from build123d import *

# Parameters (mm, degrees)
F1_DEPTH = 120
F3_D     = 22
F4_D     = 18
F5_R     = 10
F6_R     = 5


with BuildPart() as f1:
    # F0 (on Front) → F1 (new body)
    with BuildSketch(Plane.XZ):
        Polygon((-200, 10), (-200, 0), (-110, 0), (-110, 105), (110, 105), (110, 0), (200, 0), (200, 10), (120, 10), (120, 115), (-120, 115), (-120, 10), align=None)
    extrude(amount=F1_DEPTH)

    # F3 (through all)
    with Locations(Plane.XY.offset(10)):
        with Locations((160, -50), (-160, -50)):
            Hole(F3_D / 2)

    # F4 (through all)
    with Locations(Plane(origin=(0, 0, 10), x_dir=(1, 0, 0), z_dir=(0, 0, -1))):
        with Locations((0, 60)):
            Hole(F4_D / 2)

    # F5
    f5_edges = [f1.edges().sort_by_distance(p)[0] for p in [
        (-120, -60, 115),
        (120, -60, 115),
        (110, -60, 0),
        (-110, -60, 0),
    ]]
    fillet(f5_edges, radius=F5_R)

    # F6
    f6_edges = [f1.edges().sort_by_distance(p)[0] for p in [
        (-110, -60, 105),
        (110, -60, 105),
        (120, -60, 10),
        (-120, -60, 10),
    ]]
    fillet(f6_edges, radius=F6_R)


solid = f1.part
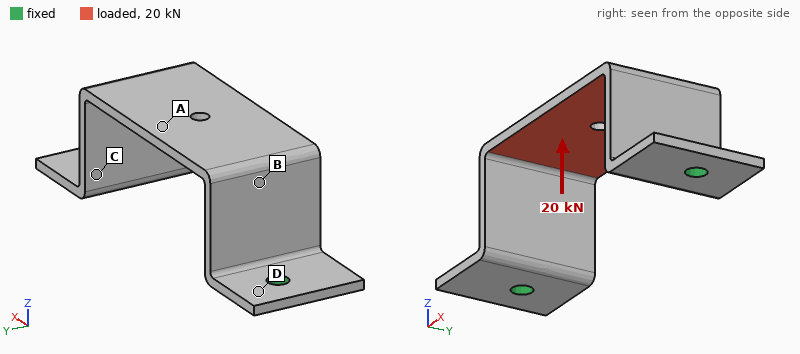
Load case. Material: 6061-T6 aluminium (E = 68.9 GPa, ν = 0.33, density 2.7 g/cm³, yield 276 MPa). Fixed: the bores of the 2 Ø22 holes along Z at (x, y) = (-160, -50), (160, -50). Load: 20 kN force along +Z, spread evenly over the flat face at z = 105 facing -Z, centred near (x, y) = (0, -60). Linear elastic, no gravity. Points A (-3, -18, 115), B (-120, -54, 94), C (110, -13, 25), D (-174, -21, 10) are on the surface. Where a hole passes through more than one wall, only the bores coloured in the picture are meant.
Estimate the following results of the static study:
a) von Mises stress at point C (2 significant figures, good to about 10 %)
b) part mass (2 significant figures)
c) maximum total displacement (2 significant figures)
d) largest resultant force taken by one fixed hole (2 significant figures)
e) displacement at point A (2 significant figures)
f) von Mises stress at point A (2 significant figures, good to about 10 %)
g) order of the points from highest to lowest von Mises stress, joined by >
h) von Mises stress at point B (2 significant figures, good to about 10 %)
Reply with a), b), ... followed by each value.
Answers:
a) 36 MPa
b) 1.9 kg
c) 1.9 mm
d) 11 kN
e) 1.6 mm
f) 140 MPa
g) A > B > C > D
h) 120 MPa
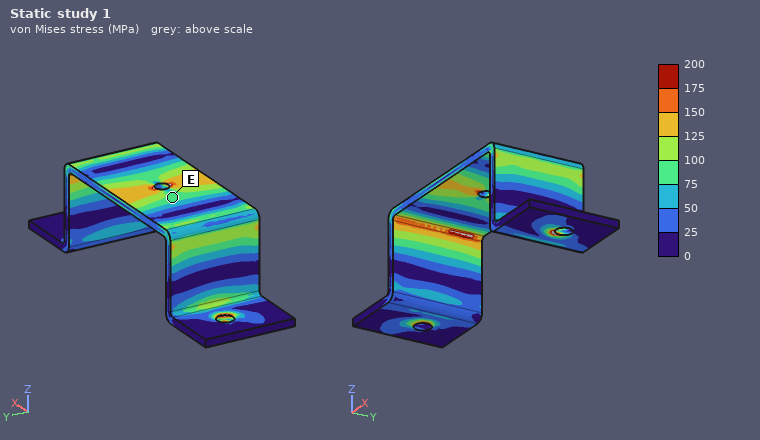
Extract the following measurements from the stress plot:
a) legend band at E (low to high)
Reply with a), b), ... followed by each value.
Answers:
a) 75 to 100 MPa
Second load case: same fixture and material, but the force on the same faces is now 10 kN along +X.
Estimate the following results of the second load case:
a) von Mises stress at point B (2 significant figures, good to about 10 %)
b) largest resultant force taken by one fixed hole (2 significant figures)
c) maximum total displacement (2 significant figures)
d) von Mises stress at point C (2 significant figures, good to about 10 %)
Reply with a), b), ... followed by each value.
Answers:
a) 85 MPa
b) 5.4 kN
c) 1.8 mm
d) 72 MPa
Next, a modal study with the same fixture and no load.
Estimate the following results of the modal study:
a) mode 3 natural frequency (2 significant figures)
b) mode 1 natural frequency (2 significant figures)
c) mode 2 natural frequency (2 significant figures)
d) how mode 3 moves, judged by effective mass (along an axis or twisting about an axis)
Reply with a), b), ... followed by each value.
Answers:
a) 570 Hz
b) 370 Hz
c) 380 Hz
d) twisting about Z
